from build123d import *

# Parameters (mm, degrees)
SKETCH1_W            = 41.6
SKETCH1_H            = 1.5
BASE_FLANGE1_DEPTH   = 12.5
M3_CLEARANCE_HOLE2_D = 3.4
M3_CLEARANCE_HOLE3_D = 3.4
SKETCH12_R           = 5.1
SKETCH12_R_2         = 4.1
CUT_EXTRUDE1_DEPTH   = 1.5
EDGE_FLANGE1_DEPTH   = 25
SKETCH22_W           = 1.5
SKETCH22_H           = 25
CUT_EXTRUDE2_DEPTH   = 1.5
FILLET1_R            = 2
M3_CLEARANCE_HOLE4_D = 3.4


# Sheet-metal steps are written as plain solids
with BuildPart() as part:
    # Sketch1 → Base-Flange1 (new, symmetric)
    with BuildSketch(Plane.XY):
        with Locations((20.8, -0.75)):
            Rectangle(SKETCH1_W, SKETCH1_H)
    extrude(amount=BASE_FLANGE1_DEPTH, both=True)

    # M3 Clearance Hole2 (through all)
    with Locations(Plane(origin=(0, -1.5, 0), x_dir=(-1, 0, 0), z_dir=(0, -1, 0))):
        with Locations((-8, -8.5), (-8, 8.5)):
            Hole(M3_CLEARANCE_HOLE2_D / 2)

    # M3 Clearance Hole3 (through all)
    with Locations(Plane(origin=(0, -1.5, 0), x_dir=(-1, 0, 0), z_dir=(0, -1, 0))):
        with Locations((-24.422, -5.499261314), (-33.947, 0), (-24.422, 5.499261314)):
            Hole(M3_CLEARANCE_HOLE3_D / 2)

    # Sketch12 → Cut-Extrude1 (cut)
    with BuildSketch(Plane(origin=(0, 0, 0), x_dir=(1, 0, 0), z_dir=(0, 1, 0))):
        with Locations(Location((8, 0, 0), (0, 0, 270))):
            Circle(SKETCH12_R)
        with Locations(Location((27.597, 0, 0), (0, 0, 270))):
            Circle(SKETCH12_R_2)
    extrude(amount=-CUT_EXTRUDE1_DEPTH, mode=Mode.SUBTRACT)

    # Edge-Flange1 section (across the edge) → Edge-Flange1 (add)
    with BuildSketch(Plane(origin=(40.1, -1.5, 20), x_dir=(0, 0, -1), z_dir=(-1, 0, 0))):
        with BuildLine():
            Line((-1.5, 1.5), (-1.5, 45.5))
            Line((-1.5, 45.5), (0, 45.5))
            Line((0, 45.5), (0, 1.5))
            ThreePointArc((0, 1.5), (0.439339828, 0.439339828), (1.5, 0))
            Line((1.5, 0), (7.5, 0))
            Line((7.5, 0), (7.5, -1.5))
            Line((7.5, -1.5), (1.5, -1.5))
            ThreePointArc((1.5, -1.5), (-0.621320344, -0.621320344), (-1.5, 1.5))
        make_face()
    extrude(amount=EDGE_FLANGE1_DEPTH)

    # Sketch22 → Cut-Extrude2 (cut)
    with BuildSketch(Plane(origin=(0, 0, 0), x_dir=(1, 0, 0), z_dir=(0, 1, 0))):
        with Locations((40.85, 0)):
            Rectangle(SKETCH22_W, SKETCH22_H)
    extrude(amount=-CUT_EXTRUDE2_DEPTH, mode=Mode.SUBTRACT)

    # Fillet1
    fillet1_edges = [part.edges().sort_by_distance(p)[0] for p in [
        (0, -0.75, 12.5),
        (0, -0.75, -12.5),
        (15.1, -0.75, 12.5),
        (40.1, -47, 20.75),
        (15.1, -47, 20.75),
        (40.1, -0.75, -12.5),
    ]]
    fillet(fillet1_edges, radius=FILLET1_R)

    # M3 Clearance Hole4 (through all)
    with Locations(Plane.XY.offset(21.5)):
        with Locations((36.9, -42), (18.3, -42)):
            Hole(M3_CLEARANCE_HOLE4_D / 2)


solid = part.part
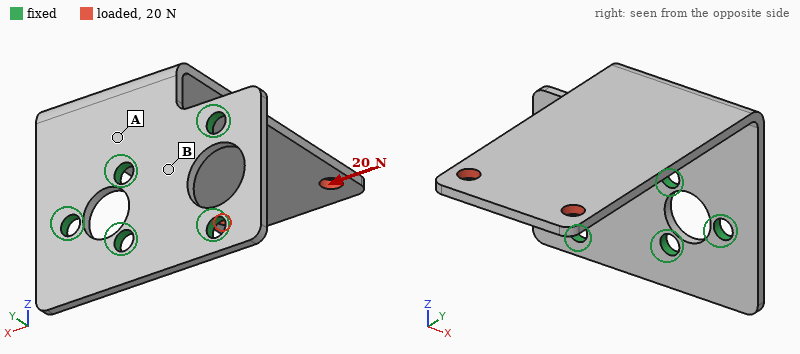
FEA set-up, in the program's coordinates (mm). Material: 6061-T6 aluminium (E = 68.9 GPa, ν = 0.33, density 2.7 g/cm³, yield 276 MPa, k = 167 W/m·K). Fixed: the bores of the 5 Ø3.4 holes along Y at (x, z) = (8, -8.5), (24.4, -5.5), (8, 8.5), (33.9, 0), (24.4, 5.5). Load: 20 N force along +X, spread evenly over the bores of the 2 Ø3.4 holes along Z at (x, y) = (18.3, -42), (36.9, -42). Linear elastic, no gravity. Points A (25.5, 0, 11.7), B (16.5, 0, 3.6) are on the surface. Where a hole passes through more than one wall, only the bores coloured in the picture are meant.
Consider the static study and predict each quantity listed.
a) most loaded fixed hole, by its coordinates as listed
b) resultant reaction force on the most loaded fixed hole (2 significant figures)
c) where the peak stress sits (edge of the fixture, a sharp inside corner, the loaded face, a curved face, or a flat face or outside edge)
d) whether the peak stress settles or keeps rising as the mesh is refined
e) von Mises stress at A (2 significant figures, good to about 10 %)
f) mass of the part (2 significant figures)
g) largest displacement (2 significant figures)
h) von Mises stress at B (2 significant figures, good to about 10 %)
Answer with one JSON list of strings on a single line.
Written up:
["(8, 8.5)", "34 N", "edge of the fixture", "keeps rising", "46 MPa", "8.7 g", "0.49 mm", "9.9 MPa"]
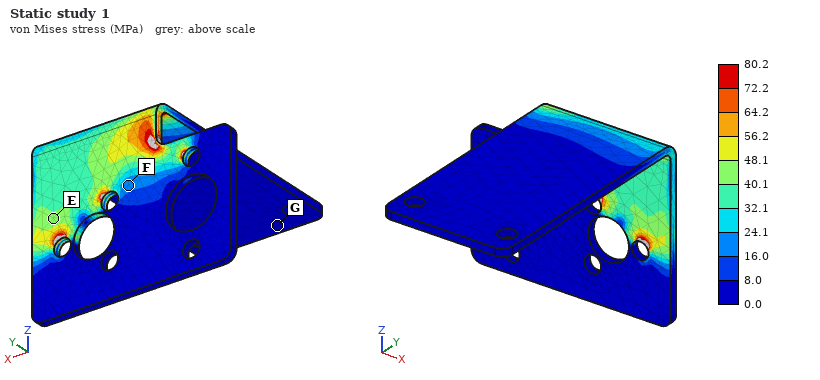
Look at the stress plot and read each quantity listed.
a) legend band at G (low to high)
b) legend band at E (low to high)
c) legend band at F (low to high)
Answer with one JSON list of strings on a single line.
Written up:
["0.0 to 8.0 MPa", "40.1 to 48.1 MPa", "16.0 to 24.1 MPa"]
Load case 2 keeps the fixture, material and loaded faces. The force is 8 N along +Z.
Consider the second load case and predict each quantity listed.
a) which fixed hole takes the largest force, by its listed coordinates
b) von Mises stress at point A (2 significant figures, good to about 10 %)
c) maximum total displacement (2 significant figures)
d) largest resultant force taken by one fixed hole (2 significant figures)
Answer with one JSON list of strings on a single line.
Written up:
["(24.4, 5.5)", "31 MPa", "0.84 mm", "12 N"]
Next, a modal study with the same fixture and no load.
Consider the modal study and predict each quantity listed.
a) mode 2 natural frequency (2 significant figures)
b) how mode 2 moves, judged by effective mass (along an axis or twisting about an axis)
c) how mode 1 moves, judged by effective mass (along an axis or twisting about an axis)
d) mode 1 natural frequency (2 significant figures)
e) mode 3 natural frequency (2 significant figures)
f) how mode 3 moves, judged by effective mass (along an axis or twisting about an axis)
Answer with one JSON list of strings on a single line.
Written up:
["800 Hz", "along X", "along Z", "400 Hz", "1900 Hz", "along Y"]
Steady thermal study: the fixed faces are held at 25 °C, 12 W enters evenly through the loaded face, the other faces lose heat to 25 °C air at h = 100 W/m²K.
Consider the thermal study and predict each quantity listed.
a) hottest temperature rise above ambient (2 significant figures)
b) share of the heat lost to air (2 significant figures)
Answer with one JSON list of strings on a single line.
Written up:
["61 K", "67 %"]
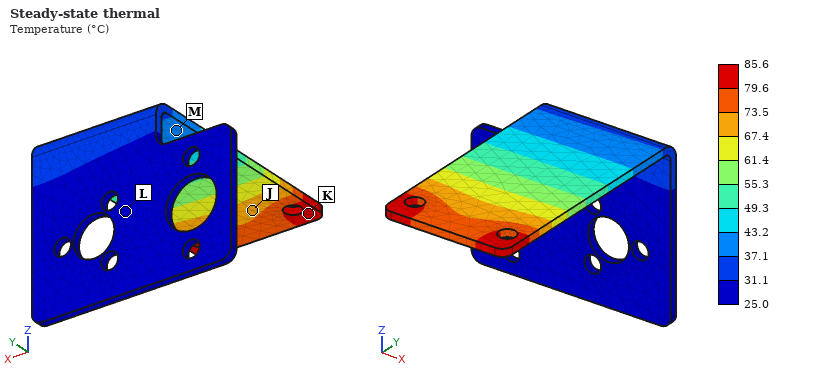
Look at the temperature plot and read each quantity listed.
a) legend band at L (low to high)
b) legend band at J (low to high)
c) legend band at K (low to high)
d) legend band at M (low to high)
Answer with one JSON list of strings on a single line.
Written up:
["25.0 to 31.1 °C", "67.4 to 73.5 °C", "79.6 to 85.6 °C", "37.1 to 43.2 °C"]
